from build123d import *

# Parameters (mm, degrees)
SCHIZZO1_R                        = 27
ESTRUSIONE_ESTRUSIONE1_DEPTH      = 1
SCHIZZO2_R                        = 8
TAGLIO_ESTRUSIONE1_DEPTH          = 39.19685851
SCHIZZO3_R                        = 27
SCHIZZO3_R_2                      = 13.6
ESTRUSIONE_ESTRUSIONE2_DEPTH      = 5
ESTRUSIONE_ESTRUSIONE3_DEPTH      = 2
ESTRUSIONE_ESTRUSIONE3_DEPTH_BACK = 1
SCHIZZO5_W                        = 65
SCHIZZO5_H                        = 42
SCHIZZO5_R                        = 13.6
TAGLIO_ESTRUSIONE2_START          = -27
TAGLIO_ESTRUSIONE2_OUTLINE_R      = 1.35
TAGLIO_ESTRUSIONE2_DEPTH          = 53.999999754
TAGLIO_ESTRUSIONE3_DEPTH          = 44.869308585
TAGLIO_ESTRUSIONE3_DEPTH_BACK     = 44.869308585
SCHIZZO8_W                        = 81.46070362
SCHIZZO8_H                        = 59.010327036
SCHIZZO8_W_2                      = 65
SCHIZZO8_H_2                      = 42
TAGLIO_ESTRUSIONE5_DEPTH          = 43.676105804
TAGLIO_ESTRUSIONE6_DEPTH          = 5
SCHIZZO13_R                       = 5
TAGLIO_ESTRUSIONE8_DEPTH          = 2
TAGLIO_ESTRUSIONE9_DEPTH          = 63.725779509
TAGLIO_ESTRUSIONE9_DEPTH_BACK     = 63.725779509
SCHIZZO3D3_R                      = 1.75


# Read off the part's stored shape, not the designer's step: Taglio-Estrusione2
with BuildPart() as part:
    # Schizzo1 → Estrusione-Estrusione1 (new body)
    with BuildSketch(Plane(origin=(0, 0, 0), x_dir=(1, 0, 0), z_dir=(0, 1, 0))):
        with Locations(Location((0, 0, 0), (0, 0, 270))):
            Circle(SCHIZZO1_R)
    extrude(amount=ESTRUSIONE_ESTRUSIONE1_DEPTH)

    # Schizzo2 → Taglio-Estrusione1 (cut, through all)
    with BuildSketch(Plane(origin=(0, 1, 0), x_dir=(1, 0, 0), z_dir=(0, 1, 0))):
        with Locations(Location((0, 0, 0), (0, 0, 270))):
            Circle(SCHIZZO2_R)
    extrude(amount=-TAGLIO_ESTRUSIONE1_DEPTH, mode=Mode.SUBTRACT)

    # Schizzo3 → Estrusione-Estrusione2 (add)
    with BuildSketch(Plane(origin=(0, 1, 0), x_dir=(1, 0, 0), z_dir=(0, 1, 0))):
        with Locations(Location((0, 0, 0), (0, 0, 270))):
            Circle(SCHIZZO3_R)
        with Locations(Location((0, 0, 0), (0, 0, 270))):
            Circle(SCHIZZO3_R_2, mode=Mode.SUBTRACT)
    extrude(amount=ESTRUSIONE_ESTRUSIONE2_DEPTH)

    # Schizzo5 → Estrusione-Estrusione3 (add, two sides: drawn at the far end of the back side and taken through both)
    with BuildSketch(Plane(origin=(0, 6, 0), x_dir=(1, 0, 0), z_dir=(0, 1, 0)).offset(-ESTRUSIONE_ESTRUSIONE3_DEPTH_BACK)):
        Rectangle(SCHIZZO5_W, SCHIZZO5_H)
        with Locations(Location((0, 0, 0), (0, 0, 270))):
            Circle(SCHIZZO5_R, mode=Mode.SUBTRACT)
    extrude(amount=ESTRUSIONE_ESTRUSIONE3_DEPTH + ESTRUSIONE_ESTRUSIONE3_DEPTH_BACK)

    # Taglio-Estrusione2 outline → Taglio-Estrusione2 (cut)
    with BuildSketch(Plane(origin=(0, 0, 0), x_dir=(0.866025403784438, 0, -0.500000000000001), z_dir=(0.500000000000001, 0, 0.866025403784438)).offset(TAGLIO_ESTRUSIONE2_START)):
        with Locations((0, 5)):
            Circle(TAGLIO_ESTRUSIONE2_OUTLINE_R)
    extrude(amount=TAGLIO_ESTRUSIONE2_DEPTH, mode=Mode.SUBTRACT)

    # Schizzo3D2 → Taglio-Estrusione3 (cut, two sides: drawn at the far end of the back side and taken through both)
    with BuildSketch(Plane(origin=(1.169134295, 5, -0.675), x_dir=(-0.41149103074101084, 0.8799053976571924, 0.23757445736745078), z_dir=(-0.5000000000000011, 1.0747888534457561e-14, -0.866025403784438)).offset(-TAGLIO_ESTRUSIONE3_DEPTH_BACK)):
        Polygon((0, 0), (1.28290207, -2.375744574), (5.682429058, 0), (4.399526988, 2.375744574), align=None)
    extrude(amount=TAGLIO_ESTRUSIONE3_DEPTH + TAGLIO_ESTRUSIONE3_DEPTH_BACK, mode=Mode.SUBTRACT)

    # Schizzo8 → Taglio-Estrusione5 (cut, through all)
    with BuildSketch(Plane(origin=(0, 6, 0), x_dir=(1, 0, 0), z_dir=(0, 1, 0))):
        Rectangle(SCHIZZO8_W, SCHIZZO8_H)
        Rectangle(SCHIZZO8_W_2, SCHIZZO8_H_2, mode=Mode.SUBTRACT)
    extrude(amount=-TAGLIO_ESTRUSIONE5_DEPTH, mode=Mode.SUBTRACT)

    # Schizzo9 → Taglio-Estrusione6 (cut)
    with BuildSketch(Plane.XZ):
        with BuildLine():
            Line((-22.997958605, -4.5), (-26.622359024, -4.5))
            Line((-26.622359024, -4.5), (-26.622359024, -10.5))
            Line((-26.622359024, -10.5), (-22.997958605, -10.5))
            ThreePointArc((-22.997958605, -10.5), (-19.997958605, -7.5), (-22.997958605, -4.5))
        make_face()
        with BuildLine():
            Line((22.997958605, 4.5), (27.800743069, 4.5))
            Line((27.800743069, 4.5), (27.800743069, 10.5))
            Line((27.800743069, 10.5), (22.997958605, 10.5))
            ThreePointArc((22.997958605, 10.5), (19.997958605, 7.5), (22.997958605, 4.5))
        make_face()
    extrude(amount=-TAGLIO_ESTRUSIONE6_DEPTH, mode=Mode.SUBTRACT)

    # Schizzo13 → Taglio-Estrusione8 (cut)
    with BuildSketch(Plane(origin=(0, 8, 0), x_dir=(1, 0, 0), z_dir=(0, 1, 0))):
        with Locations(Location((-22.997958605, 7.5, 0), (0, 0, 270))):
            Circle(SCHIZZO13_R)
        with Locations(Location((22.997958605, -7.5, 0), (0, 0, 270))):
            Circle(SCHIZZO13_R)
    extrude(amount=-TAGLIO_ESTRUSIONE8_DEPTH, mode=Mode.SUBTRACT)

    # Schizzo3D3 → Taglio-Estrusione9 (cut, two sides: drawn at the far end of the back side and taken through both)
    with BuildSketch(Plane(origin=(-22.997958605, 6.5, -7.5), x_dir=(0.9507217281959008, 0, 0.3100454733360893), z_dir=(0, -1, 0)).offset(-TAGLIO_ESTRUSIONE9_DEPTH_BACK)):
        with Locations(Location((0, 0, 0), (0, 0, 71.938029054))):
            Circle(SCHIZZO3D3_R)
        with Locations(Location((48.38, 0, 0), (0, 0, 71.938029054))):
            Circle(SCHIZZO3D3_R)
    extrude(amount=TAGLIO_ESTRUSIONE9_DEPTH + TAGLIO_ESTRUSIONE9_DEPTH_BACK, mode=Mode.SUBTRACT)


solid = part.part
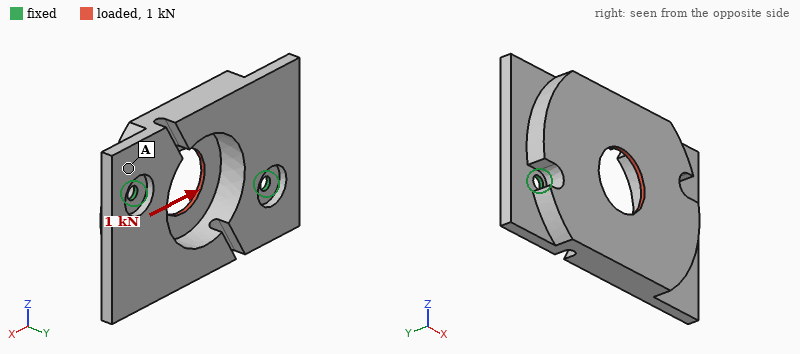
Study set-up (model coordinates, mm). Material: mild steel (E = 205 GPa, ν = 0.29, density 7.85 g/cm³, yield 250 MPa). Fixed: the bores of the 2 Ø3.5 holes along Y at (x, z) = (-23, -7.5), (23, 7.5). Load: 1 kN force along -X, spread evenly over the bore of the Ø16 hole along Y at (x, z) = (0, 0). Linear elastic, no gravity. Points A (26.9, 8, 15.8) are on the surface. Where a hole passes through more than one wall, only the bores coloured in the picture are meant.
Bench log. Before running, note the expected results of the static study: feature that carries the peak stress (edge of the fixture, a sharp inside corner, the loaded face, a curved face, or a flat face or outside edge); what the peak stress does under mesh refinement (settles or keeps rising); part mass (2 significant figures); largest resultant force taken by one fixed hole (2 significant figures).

edge of the fixture
keeps rising
100 g
510 N
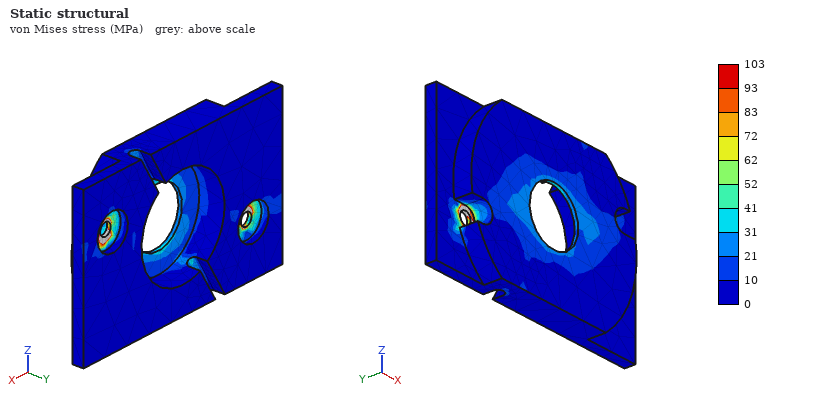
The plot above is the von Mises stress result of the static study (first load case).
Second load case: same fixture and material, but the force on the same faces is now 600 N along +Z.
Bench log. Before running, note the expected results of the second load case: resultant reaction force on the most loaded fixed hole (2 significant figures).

300 N
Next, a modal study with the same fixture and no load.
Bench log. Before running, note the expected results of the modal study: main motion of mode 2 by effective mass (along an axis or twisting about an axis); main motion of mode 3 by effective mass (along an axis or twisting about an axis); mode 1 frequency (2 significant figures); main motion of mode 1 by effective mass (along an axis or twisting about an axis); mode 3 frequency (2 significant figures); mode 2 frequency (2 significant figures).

along Y
along Y
1400 Hz
twisting about X
6800 Hz
5100 Hz
